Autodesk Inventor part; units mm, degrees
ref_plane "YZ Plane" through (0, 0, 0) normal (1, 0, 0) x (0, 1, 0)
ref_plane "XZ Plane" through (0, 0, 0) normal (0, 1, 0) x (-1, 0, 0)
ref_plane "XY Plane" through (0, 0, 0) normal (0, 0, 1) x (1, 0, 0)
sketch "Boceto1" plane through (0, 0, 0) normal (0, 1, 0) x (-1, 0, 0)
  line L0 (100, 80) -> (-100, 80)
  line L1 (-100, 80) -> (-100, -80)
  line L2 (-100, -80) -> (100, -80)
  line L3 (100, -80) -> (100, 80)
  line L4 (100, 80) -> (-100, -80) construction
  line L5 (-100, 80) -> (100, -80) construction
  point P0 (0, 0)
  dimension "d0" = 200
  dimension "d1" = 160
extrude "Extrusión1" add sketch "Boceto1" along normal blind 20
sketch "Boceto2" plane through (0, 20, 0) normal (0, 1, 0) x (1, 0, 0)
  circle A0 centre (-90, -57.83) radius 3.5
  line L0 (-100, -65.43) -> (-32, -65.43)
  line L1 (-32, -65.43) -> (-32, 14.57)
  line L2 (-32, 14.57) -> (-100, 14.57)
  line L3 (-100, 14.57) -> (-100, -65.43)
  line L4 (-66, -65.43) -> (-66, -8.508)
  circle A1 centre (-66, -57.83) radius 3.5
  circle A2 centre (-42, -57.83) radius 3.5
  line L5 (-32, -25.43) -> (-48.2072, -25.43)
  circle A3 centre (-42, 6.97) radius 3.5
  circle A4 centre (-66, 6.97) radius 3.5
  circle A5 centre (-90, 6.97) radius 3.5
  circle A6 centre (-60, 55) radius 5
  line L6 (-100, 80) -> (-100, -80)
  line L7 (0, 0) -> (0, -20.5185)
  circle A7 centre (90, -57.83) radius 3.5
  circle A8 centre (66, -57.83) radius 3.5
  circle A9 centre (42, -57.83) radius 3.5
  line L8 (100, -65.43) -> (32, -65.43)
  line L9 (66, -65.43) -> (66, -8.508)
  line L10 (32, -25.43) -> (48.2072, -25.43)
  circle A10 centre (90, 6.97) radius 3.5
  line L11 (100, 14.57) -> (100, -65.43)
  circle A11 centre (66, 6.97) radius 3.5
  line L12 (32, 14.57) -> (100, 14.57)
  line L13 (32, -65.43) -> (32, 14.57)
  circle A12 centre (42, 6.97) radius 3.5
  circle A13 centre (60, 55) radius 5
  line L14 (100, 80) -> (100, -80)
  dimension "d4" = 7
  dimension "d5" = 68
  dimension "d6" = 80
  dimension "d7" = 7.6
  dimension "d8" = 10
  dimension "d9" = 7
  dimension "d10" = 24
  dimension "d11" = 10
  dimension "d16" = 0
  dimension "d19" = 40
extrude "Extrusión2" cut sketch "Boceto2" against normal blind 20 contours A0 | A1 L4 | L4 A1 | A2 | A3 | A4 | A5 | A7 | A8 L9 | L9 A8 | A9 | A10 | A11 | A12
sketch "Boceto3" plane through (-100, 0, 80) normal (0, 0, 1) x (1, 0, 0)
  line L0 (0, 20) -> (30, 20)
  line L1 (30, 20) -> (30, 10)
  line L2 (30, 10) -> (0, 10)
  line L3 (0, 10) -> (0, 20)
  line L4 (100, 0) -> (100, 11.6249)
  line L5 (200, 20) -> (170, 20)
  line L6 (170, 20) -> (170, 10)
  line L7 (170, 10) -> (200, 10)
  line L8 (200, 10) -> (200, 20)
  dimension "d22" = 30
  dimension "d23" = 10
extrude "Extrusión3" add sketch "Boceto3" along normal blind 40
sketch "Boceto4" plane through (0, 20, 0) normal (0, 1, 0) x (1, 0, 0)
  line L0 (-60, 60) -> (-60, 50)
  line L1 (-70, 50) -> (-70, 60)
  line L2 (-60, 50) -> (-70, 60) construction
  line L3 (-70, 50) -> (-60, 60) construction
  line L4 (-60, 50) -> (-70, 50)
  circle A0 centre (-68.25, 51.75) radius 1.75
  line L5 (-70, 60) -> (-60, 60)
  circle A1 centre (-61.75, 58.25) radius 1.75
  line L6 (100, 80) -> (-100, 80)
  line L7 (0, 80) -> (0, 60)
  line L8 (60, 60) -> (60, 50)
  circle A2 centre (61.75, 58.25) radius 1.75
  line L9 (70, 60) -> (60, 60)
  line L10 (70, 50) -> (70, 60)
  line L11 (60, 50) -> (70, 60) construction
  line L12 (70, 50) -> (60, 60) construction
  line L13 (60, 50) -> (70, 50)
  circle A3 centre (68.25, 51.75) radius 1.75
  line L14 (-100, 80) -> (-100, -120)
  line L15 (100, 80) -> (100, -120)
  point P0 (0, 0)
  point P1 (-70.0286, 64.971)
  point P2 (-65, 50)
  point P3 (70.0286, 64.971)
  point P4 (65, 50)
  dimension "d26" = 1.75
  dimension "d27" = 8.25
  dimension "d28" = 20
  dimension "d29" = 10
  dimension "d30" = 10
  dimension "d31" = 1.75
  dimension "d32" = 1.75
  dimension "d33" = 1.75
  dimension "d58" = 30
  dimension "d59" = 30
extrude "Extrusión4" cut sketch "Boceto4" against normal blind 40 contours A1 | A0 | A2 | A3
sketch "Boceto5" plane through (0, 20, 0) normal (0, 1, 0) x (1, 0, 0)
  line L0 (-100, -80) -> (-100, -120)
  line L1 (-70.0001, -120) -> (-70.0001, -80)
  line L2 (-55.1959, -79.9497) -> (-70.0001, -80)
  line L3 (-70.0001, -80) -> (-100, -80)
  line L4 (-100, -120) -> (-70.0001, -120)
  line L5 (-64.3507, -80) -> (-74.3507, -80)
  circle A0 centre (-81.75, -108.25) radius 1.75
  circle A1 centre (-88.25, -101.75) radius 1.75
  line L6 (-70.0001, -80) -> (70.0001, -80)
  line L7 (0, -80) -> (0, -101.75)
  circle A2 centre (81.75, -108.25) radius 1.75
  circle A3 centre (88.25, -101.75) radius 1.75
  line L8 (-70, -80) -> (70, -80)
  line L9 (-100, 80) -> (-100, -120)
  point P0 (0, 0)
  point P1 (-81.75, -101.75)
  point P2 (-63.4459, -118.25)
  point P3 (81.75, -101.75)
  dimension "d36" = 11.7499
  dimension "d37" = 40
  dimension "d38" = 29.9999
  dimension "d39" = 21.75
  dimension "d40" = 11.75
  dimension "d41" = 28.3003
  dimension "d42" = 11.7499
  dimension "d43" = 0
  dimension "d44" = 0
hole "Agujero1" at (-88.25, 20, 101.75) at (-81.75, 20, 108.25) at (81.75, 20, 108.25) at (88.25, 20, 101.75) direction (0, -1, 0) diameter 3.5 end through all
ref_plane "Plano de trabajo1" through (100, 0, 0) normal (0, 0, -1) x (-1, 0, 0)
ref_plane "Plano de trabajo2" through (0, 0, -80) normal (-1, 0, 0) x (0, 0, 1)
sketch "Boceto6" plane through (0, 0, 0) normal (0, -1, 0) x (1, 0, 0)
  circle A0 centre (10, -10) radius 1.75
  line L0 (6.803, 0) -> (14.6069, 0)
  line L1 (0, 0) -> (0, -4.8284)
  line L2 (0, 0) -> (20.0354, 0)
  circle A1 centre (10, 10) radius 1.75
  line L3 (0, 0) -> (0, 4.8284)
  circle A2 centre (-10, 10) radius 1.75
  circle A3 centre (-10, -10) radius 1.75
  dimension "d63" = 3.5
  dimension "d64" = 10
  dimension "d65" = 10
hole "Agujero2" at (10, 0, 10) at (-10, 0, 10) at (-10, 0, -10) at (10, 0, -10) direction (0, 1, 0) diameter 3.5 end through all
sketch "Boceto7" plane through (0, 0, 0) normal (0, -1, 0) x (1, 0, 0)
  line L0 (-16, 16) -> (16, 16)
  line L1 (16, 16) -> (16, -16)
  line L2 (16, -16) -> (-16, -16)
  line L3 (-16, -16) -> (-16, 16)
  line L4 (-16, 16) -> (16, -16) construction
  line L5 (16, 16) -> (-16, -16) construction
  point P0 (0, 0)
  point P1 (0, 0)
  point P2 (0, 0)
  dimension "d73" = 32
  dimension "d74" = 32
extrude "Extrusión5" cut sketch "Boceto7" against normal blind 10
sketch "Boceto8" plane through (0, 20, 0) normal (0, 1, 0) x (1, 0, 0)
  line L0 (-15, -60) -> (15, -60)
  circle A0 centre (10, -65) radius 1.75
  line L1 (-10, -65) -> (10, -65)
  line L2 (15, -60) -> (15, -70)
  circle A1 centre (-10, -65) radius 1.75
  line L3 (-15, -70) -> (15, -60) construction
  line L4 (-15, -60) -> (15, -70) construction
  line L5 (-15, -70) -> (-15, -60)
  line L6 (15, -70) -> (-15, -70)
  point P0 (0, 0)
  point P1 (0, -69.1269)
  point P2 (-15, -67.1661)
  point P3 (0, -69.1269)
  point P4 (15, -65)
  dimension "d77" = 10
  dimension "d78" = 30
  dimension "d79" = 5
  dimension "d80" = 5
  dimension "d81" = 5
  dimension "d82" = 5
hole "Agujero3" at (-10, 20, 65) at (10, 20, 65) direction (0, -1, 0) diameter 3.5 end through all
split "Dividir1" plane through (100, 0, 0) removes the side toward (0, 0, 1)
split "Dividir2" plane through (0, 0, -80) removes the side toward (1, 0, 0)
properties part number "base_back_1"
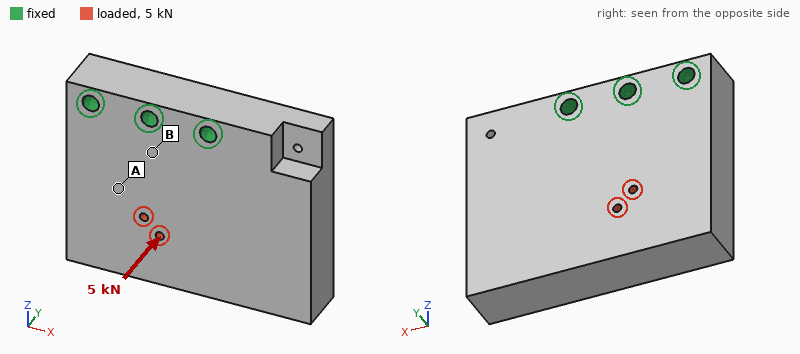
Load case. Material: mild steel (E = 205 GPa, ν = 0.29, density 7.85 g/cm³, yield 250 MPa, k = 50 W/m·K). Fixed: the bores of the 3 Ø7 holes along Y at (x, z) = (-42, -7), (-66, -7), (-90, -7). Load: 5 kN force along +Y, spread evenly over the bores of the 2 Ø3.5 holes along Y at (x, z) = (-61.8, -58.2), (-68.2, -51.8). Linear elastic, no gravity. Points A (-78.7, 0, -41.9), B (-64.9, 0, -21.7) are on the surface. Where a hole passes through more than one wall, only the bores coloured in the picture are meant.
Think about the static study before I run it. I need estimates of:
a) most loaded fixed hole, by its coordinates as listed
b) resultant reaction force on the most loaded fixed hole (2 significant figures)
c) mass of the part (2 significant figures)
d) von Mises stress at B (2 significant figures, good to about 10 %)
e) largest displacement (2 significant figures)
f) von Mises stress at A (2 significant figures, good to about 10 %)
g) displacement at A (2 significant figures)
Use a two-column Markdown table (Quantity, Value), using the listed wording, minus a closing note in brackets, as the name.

| Quantity | Value |
|---|---|
| most loaded fixed hole, by its coordinates as listed | (-66, -7) |
| resultant reaction force on the most loaded fixed hole | 2.3 kN |
| mass of the part | 1.2 kg |
| von Mises stress at B | 33 MPa |
| largest displacement | 35 µm |
| von Mises stress at A | 13 MPa |
| displacement at A | 14 µm |
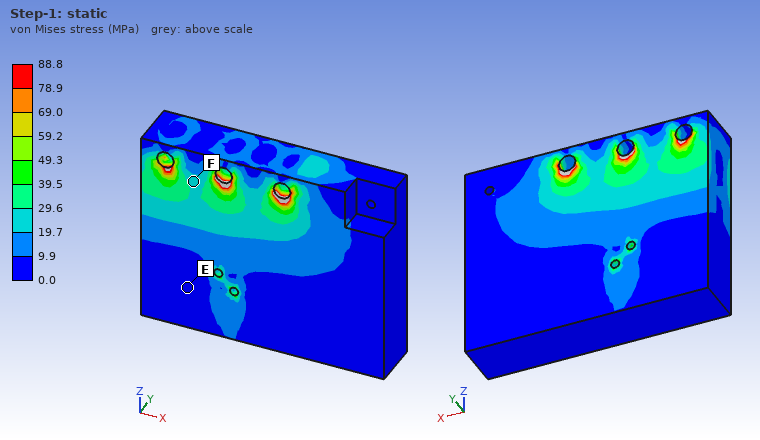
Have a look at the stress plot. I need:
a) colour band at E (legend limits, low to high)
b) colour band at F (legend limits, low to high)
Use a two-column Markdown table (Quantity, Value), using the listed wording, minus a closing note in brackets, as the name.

| Quantity | Value |
|---|---|
| colour band at E | 0.0 to 9.9 MPa |
| colour band at F | 19.7 to 29.6 MPa |
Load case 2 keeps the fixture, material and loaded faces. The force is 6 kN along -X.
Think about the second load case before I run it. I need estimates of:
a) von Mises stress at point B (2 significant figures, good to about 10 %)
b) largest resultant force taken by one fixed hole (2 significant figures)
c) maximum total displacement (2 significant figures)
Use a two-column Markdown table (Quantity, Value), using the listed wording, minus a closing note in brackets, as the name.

| Quantity | Value |
|---|---|
| von Mises stress at point B | 9.7 MPa |
| largest resultant force taken by one fixed hole | 5.7 kN |
| maximum total displacement | 8.2 µm |
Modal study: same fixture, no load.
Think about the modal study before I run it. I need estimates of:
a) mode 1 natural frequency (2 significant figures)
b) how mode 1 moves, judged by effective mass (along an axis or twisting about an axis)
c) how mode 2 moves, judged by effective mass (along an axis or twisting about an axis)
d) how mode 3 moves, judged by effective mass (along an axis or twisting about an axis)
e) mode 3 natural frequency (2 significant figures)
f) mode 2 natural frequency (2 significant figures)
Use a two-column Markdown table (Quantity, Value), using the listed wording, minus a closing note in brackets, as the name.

| Quantity | Value |
|---|---|
| mode 1 natural frequency | 2500 Hz |
| how mode 1 moves, judged by effective mass | along Y |
| how mode 2 moves, judged by effective mass | twisting about Z |
| how mode 3 moves, judged by effective mass | along X |
| mode 3 natural frequency | 5200 Hz |
| mode 2 natural frequency | 4300 Hz |
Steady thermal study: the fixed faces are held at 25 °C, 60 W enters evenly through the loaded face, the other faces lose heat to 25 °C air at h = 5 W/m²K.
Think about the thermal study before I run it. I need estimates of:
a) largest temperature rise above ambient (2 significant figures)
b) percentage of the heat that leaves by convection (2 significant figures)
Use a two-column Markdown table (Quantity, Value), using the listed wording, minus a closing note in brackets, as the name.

| Quantity | Value |
|---|---|
| largest temperature rise above ambient | 48 K |
| percentage of the heat that leaves by convection | 3.8 % |
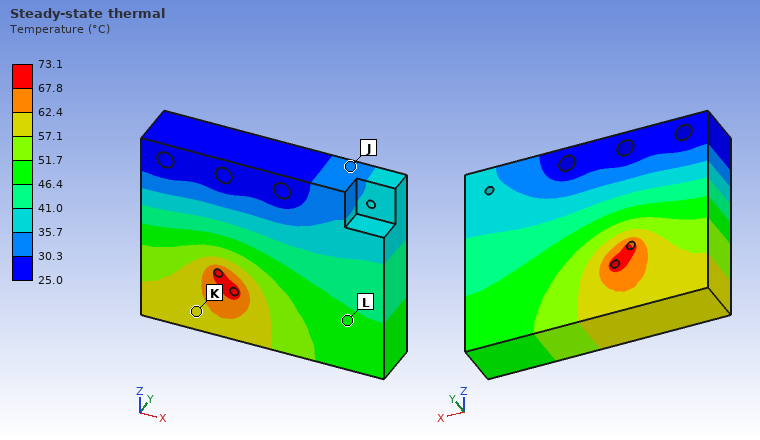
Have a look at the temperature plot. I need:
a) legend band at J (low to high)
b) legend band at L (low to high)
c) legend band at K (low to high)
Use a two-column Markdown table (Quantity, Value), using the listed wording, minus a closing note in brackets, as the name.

| Quantity | Value |
|---|---|
| legend band at J | 30.3 to 35.7 °C |
| legend band at L | 46.4 to 51.7 °C |
| legend band at K | 57.1 to 62.4 °C |
